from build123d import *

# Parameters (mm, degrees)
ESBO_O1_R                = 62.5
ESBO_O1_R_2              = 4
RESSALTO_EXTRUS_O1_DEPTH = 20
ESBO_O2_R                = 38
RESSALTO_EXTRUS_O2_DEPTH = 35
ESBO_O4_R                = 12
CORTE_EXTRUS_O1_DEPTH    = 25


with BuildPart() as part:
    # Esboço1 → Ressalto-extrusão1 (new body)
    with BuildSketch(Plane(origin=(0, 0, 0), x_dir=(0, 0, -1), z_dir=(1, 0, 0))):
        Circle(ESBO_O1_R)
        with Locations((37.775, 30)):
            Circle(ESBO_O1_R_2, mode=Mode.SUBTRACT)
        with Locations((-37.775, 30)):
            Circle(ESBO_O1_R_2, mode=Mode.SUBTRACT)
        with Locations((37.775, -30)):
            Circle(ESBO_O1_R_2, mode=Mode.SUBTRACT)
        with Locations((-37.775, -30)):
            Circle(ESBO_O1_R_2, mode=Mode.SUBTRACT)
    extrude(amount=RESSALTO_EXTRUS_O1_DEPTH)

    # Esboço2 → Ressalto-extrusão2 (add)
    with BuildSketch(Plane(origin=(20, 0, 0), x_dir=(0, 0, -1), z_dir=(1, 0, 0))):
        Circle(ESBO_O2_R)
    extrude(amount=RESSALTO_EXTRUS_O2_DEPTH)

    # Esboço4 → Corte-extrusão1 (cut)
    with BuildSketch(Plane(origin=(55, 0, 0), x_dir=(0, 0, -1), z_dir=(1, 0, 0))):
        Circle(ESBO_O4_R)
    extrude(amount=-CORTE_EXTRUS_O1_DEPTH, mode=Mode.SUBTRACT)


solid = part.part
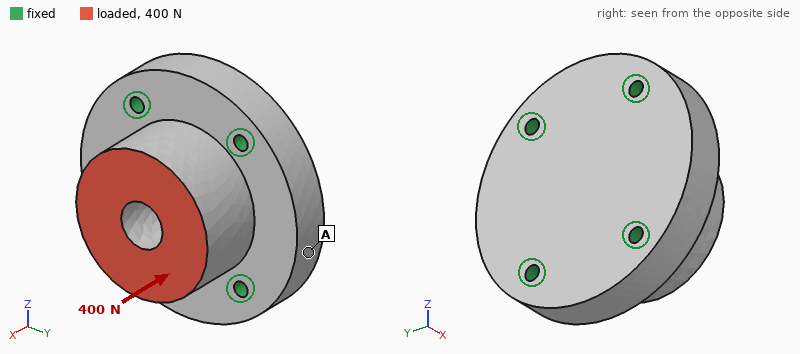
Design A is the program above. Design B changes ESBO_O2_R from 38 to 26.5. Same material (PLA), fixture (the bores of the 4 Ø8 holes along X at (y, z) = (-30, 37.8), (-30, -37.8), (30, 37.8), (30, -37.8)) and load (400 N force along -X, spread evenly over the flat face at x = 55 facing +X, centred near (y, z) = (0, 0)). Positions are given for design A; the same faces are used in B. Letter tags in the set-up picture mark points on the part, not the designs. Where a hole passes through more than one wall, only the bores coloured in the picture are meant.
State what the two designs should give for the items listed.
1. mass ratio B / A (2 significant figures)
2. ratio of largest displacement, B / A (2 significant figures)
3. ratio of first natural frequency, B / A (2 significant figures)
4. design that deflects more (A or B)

0.79
2.0
1.0
B
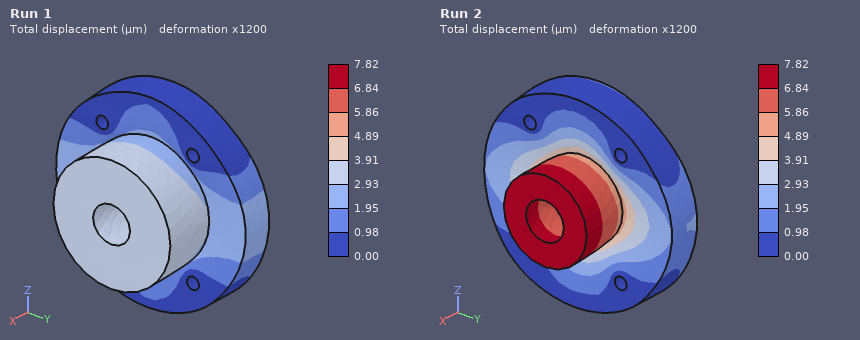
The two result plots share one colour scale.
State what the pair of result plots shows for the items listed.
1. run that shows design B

Run 2
